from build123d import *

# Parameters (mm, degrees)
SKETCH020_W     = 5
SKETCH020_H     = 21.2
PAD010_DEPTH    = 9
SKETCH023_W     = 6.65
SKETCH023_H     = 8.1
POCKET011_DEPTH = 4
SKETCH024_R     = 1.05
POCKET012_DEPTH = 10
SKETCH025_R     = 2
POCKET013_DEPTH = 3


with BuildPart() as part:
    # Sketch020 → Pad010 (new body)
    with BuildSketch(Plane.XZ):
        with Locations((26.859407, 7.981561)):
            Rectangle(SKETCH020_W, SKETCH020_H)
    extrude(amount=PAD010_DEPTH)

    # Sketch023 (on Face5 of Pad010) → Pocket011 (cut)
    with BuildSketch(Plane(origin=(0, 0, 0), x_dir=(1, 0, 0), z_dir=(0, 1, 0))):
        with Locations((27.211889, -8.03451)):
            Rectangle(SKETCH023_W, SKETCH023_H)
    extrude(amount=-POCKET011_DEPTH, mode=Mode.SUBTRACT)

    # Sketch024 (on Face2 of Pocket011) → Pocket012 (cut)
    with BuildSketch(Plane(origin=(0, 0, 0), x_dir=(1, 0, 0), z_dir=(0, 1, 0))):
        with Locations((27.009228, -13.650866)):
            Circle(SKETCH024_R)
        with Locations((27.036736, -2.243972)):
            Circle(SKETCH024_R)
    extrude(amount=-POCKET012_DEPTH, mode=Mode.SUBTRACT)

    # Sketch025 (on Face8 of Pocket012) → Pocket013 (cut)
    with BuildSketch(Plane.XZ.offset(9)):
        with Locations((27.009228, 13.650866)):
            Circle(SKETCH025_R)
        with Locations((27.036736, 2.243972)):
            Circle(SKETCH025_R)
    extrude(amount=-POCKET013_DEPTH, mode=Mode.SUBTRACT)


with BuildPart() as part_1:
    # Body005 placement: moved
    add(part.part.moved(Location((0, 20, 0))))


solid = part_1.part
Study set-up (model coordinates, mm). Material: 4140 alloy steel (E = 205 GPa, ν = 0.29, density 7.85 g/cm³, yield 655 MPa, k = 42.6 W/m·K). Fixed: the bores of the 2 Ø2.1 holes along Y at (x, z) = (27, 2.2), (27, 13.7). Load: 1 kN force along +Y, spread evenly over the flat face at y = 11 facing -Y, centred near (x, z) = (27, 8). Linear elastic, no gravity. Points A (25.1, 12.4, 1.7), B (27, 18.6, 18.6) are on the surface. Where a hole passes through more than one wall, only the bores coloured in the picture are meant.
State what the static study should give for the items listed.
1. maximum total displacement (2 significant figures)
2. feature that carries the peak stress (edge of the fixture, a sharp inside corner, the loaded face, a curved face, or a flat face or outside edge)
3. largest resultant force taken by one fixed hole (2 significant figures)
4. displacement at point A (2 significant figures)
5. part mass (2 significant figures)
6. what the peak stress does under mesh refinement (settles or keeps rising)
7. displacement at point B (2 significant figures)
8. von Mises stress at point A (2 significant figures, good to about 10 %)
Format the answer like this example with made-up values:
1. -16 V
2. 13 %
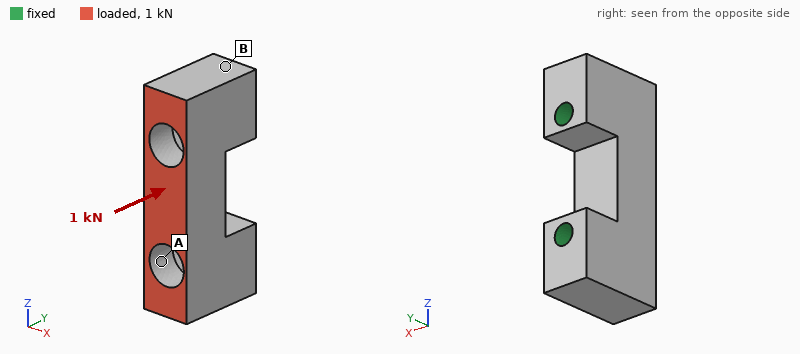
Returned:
1. 1.1 µm
2. edge of the fixture
3. 510 N
4. 0.44 µm
5. 5.3 g
6. keeps rising
7. 0.36 µm
8. 23 MPa
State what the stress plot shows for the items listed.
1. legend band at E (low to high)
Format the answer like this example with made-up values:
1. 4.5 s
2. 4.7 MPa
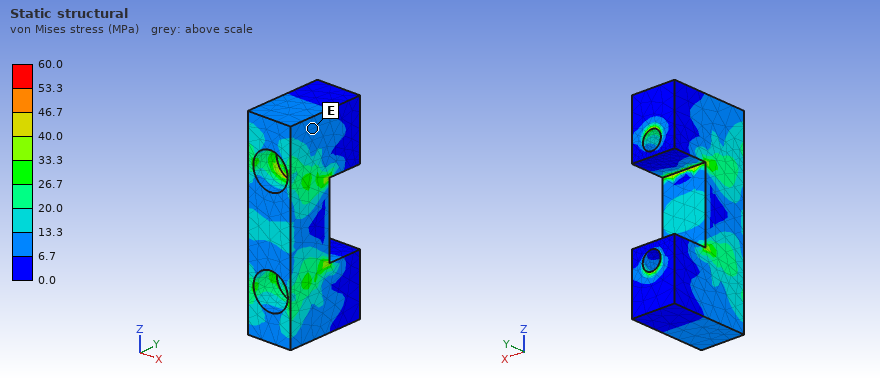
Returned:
1. 6.7 to 13.3 MPa
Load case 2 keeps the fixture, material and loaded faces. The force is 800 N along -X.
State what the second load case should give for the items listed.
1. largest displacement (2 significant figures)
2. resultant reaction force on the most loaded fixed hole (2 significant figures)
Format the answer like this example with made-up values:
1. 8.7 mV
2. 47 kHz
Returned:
1. 5.0 µm
2. 400 N
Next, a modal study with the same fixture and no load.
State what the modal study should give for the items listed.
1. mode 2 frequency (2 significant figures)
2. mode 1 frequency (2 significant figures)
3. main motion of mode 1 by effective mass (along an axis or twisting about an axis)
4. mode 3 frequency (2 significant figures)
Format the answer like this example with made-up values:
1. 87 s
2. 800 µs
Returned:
1. 75 kHz
2. 64 kHz
3. along X
4. 76 kHz
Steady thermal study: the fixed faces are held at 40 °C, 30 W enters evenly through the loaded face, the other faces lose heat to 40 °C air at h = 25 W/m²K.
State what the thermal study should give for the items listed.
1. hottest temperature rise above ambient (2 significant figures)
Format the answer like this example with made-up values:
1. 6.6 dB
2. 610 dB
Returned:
1. 64 K
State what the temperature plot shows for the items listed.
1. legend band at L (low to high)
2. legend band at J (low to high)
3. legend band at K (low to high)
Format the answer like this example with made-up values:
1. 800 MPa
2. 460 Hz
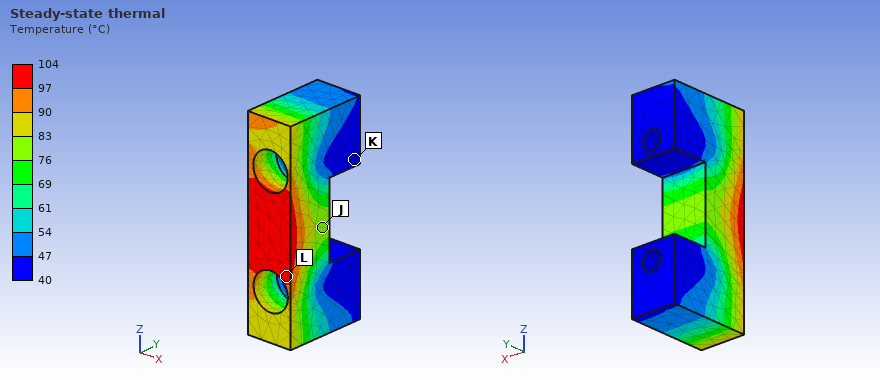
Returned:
1. 97 to 104 °C
2. 76 to 83 °C
3. 40 to 47 °C
